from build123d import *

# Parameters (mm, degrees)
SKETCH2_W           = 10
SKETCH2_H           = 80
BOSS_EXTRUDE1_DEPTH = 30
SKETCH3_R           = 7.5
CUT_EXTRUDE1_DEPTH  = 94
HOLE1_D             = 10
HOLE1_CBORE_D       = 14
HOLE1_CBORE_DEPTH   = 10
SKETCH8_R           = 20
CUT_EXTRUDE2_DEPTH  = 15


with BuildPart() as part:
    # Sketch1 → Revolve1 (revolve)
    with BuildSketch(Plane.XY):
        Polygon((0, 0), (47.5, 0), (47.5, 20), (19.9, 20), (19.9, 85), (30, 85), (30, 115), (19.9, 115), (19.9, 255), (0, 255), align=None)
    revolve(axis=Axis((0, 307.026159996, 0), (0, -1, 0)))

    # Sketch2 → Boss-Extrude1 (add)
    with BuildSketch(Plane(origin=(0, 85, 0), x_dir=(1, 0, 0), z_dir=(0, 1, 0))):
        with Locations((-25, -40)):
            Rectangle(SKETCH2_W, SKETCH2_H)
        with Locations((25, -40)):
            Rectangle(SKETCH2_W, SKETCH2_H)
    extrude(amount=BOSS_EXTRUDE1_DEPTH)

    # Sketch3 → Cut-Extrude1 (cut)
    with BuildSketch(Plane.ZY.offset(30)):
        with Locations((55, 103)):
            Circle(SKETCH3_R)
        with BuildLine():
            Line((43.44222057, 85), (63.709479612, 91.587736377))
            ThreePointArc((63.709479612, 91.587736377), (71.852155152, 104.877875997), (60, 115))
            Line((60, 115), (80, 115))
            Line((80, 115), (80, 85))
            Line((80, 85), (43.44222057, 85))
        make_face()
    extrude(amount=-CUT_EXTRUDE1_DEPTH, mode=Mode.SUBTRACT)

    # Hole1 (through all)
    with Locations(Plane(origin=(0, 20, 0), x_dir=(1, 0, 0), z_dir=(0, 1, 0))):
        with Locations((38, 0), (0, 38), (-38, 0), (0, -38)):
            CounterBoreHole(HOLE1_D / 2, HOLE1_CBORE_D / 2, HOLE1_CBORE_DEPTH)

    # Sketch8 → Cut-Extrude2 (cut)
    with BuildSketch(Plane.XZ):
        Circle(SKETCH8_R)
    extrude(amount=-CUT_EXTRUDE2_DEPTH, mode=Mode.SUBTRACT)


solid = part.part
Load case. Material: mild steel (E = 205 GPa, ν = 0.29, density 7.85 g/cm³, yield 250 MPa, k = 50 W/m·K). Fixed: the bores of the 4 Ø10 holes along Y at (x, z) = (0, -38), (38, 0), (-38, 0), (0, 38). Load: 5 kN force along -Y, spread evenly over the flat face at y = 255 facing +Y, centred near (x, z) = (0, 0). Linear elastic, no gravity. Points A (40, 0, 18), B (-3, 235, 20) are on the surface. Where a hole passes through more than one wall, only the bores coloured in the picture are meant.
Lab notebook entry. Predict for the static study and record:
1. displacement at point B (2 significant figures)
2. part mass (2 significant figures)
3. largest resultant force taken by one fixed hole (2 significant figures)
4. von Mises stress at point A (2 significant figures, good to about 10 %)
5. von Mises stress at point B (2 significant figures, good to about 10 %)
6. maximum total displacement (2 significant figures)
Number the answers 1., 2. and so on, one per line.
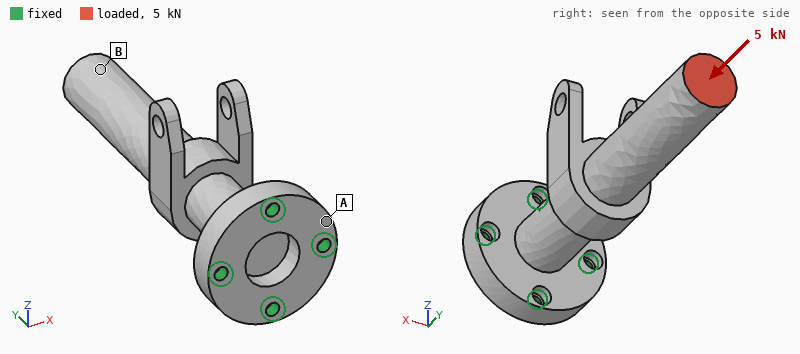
1. 5.5 µm
2. 3.8 kg
3. 1.5 kN
4. 2.1 MPa
5. 4.0 MPa
6. 5.9 µm
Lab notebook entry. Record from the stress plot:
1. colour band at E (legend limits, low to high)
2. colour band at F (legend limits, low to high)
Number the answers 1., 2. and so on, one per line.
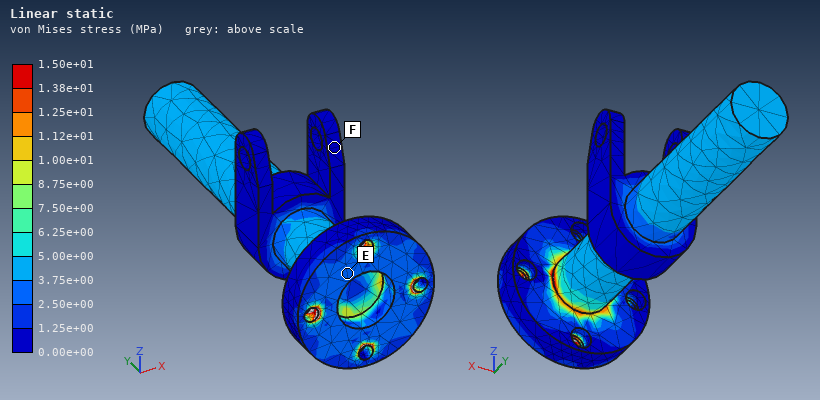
1. 2.50e+00 to 3.75e+00 MPa
2. 0.00e+00 to 1.25e+00 MPa
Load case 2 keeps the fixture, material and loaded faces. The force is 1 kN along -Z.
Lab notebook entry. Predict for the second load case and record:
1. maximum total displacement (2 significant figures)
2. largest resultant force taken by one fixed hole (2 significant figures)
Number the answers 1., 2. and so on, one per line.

1. 0.22 mm
2. 4.0 kN
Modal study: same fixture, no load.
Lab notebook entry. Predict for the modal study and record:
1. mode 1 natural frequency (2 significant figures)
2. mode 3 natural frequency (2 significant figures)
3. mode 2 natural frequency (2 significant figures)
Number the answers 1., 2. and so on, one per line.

1. 420 Hz
2. 2000 Hz
3. 420 Hz
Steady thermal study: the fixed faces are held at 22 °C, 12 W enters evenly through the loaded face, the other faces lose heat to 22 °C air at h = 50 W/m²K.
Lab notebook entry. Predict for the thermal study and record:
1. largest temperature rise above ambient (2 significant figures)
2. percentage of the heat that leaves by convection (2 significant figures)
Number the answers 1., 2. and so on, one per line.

1. 19 K
2. 89 %
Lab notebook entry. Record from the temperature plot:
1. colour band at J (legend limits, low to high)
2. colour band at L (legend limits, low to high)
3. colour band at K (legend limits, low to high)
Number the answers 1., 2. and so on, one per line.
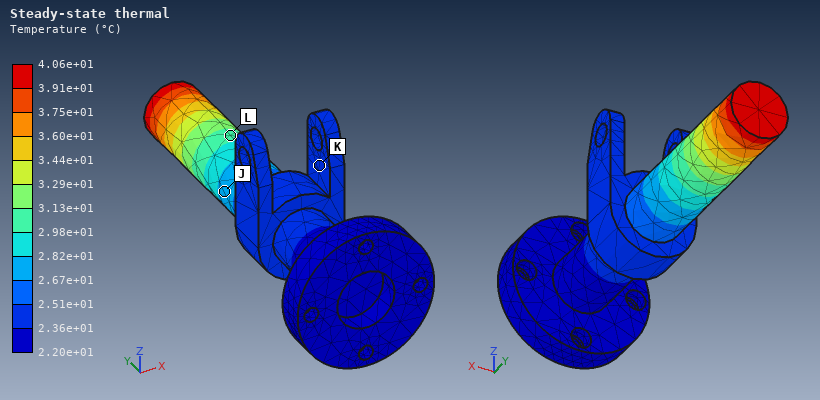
1. 2.67e+01 to 2.82e+01 °C
2. 2.98e+01 to 3.13e+01 °C
3. 2.36e+01 to 2.51e+01 °C
